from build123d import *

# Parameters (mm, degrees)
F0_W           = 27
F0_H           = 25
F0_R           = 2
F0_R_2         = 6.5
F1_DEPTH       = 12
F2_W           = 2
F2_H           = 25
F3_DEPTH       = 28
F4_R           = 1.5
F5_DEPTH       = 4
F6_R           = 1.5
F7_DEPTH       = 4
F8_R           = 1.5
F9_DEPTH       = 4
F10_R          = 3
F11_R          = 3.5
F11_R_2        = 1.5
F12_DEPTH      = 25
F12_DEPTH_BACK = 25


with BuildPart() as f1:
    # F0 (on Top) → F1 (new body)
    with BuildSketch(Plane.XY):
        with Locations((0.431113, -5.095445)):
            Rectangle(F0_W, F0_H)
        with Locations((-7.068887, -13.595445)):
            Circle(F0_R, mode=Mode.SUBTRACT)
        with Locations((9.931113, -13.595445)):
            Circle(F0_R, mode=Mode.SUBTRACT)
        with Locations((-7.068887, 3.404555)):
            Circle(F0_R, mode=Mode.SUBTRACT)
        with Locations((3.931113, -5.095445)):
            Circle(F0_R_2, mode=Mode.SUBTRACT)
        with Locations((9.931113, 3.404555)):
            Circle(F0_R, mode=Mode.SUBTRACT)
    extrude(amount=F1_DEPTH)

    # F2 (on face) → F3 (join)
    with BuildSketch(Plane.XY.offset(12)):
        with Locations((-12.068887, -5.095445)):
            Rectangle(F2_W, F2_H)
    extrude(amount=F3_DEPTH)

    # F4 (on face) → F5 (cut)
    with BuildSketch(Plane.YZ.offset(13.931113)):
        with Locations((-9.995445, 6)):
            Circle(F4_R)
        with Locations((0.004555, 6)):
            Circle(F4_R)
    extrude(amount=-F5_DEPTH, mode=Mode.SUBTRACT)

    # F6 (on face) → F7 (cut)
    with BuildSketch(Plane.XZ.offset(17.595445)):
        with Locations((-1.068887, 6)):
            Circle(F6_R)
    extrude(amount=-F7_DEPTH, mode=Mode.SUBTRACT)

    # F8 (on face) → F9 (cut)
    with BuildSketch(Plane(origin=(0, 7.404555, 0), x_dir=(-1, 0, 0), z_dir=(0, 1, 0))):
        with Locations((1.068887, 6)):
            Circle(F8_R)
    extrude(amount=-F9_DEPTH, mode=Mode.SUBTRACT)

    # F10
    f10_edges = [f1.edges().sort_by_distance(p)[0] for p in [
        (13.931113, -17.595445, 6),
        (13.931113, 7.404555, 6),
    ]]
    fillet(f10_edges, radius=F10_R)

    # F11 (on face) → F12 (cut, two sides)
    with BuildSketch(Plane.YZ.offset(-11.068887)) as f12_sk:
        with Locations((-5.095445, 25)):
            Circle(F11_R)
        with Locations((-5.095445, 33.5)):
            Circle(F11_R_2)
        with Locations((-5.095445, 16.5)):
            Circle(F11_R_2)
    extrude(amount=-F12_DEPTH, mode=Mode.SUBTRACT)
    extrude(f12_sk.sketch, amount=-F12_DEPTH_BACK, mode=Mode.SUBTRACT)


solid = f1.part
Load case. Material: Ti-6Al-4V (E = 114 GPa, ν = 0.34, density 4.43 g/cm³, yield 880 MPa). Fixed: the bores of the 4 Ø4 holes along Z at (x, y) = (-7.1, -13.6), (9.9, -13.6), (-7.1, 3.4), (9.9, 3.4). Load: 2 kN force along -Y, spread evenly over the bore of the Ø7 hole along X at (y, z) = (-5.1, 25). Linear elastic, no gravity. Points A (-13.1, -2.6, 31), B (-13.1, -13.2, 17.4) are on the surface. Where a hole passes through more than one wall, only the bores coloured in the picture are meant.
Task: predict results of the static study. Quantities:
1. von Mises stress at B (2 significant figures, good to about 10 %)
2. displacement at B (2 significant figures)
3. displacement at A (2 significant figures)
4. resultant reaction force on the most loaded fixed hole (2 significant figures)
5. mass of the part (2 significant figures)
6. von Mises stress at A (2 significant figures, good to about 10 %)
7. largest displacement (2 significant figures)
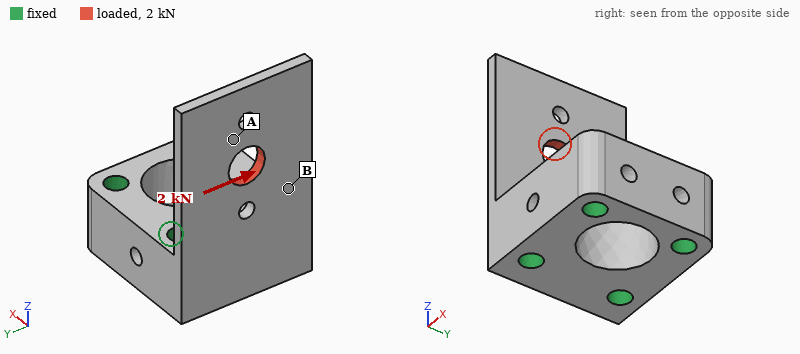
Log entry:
74 MPa
15 µm
42 µm
1.9 kN
31 g
27 MPa
57 µm
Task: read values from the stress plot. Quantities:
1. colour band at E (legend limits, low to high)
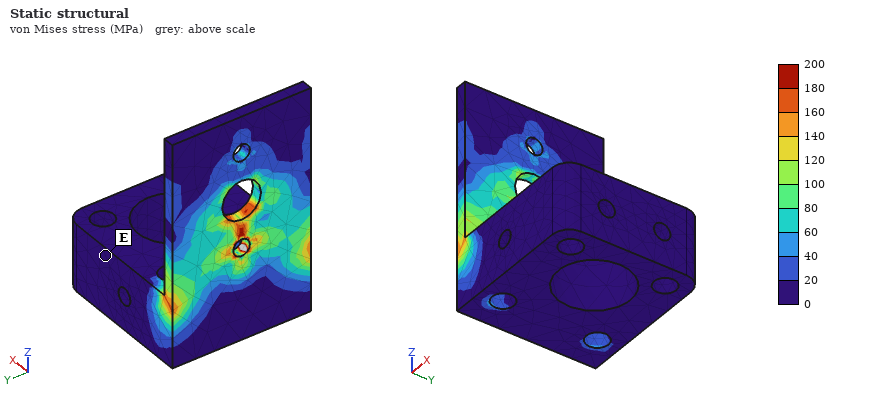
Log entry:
0 to 20 MPa
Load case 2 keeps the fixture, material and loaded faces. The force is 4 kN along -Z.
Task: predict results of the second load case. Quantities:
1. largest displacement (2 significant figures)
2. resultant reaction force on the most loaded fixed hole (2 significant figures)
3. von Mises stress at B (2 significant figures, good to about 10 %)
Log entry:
38 µm
2.1 kN
81 MPa
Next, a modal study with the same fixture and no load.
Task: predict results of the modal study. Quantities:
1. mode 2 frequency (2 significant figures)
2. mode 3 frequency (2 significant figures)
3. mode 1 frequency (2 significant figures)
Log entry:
5000 Hz
12 kHz
1900 Hz
